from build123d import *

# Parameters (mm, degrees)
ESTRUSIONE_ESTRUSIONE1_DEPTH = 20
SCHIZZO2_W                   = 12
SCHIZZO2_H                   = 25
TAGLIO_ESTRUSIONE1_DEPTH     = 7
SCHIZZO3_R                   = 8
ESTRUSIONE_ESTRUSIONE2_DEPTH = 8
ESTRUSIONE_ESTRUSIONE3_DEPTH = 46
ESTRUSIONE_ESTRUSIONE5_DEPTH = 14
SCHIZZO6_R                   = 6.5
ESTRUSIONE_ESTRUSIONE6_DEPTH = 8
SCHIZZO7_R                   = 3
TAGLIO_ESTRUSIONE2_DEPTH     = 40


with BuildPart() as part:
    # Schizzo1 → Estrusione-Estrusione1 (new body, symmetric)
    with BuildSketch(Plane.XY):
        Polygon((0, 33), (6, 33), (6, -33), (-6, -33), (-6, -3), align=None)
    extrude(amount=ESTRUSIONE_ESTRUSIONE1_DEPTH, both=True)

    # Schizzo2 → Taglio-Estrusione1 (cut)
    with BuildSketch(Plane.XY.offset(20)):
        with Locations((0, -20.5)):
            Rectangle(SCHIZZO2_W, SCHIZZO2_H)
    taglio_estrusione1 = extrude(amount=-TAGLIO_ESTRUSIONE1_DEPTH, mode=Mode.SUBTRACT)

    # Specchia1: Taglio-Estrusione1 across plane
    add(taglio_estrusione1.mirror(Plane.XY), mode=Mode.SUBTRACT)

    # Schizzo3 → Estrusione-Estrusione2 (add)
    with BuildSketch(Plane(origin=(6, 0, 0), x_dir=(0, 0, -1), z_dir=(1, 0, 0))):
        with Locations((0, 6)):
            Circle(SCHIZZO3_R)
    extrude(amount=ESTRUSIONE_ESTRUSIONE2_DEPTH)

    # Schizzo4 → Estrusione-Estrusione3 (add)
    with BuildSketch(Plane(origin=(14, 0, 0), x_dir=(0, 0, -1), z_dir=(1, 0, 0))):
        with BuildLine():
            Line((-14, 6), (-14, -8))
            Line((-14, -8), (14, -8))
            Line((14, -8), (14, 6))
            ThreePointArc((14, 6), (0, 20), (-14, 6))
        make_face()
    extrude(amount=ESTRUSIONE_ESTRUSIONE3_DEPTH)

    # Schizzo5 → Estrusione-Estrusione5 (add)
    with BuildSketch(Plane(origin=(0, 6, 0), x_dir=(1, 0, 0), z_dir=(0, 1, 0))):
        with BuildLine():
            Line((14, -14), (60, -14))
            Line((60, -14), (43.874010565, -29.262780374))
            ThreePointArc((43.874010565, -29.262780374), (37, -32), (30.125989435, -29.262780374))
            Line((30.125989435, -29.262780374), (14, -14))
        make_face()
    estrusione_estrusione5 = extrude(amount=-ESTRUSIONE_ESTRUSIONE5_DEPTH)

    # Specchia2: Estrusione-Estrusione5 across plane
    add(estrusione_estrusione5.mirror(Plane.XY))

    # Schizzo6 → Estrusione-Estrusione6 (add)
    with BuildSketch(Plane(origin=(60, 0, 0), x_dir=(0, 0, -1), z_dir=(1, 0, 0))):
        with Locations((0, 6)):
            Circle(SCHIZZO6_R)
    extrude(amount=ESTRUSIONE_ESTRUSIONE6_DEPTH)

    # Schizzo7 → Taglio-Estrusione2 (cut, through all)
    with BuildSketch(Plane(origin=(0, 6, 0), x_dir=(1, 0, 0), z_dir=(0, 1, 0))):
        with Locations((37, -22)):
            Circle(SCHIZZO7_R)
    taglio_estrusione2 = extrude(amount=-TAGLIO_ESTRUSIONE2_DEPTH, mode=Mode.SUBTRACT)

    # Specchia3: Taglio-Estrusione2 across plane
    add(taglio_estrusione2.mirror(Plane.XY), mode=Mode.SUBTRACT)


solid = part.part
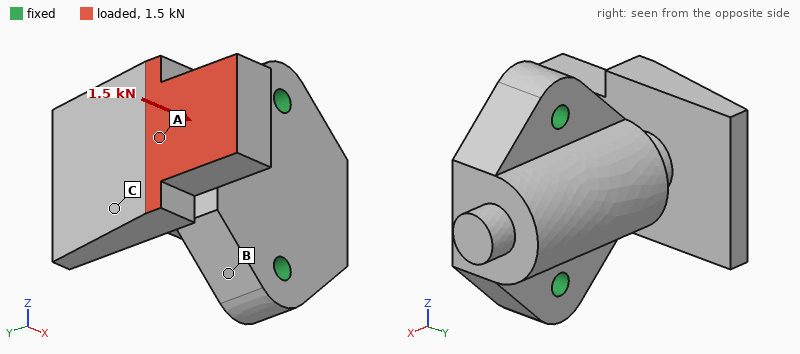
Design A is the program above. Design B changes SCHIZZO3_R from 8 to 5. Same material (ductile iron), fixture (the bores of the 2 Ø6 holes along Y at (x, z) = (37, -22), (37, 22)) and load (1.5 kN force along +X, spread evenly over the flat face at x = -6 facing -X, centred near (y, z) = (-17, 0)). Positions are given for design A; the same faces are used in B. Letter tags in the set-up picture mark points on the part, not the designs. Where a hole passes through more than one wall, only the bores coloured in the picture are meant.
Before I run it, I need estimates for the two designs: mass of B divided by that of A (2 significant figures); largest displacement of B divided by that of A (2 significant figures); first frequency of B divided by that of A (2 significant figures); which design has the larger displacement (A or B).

0.99
3.9
0.52
B
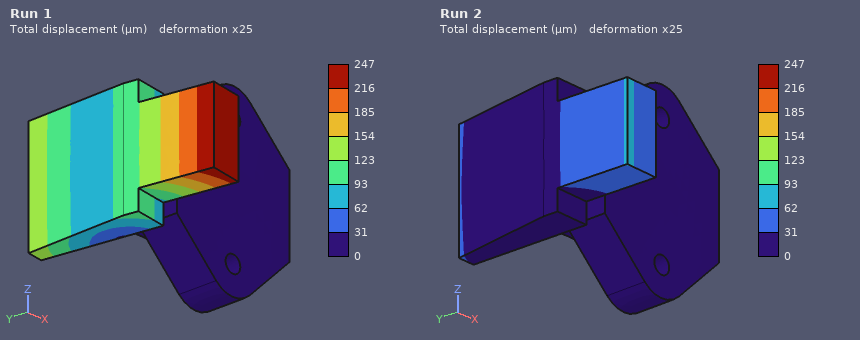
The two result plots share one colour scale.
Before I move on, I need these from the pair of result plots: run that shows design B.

Run 1
